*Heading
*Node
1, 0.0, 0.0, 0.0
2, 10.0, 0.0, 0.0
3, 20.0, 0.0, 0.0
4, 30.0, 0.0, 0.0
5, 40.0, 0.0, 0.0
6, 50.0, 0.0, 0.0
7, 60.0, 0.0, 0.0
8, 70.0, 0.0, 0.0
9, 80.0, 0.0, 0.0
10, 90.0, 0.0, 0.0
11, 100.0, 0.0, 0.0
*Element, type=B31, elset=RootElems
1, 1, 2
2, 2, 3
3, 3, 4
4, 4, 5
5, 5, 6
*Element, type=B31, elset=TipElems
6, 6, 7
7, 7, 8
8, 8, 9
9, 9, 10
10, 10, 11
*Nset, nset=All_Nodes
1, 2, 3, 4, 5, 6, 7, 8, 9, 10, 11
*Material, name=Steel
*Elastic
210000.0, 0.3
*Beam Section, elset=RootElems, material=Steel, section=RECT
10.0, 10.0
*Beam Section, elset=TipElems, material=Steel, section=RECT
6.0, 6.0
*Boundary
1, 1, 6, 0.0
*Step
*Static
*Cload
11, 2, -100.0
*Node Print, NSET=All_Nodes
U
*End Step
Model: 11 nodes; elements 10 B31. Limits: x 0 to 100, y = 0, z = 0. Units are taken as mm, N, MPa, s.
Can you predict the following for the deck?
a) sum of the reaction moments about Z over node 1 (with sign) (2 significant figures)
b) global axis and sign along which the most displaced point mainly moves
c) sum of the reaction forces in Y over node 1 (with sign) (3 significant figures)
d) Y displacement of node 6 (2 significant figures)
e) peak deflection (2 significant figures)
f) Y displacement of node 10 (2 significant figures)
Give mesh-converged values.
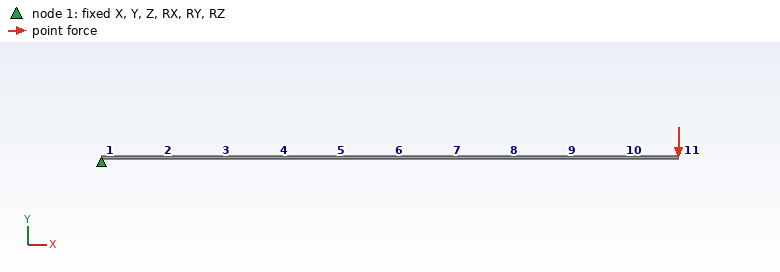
10000 N·mm
-Y
100 N
-0.060 mm
0.35 mm
-0.28 mm
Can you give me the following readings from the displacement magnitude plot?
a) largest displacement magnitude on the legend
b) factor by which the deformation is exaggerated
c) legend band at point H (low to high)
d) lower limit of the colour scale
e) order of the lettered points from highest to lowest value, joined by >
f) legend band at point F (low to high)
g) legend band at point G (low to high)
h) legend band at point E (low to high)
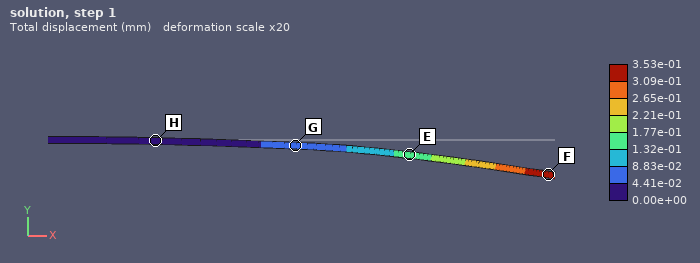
3.53e-01 mm
20
0.00e+00 to 4.41e-02 mm
0.00e+00 mm
F > E > G > H
3.09e-01 to 3.53e-01 mm
4.41e-02 to 8.83e-02 mm
1.32e-01 to 1.77e-01 mm
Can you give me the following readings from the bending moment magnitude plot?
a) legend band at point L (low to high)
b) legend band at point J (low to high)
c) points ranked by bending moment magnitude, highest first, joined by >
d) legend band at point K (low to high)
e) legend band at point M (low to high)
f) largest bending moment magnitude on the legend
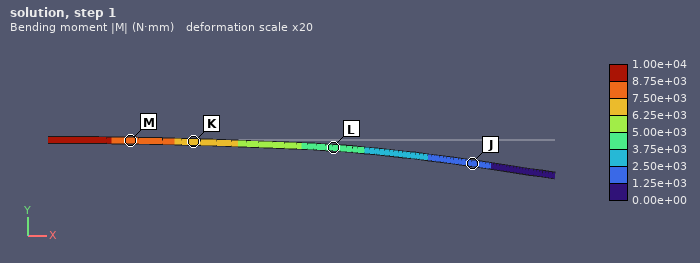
3.75e+03 to 5.00e+03 N·mm
1.25e+03 to 2.50e+03 N·mm
M > K > L > J
6.25e+03 to 7.50e+03 N·mm
7.50e+03 to 8.75e+03 N·mm
1.00e+04 N·mm
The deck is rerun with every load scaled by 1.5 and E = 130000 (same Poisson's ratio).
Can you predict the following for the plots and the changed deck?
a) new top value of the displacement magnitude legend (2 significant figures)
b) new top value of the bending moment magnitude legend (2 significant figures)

0.86 mm
15000 N·mm
